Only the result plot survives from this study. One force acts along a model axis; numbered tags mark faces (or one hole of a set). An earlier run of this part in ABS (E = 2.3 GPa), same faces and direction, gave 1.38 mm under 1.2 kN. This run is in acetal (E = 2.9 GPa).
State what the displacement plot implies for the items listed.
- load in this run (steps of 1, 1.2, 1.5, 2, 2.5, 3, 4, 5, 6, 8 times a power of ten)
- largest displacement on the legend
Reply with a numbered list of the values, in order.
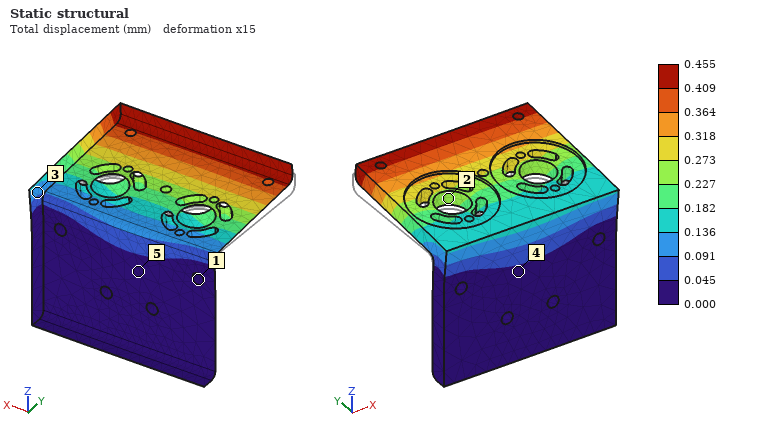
1. 500 N
2. 0.455 mm
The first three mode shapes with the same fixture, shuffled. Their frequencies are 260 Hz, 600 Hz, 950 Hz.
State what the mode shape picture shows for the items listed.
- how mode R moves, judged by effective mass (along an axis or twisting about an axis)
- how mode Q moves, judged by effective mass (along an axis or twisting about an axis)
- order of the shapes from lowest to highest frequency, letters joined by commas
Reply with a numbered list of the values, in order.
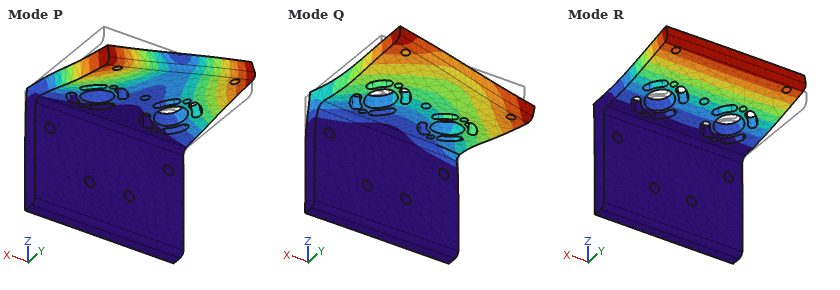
1. along Z
2. along X
3. R, P, Q
